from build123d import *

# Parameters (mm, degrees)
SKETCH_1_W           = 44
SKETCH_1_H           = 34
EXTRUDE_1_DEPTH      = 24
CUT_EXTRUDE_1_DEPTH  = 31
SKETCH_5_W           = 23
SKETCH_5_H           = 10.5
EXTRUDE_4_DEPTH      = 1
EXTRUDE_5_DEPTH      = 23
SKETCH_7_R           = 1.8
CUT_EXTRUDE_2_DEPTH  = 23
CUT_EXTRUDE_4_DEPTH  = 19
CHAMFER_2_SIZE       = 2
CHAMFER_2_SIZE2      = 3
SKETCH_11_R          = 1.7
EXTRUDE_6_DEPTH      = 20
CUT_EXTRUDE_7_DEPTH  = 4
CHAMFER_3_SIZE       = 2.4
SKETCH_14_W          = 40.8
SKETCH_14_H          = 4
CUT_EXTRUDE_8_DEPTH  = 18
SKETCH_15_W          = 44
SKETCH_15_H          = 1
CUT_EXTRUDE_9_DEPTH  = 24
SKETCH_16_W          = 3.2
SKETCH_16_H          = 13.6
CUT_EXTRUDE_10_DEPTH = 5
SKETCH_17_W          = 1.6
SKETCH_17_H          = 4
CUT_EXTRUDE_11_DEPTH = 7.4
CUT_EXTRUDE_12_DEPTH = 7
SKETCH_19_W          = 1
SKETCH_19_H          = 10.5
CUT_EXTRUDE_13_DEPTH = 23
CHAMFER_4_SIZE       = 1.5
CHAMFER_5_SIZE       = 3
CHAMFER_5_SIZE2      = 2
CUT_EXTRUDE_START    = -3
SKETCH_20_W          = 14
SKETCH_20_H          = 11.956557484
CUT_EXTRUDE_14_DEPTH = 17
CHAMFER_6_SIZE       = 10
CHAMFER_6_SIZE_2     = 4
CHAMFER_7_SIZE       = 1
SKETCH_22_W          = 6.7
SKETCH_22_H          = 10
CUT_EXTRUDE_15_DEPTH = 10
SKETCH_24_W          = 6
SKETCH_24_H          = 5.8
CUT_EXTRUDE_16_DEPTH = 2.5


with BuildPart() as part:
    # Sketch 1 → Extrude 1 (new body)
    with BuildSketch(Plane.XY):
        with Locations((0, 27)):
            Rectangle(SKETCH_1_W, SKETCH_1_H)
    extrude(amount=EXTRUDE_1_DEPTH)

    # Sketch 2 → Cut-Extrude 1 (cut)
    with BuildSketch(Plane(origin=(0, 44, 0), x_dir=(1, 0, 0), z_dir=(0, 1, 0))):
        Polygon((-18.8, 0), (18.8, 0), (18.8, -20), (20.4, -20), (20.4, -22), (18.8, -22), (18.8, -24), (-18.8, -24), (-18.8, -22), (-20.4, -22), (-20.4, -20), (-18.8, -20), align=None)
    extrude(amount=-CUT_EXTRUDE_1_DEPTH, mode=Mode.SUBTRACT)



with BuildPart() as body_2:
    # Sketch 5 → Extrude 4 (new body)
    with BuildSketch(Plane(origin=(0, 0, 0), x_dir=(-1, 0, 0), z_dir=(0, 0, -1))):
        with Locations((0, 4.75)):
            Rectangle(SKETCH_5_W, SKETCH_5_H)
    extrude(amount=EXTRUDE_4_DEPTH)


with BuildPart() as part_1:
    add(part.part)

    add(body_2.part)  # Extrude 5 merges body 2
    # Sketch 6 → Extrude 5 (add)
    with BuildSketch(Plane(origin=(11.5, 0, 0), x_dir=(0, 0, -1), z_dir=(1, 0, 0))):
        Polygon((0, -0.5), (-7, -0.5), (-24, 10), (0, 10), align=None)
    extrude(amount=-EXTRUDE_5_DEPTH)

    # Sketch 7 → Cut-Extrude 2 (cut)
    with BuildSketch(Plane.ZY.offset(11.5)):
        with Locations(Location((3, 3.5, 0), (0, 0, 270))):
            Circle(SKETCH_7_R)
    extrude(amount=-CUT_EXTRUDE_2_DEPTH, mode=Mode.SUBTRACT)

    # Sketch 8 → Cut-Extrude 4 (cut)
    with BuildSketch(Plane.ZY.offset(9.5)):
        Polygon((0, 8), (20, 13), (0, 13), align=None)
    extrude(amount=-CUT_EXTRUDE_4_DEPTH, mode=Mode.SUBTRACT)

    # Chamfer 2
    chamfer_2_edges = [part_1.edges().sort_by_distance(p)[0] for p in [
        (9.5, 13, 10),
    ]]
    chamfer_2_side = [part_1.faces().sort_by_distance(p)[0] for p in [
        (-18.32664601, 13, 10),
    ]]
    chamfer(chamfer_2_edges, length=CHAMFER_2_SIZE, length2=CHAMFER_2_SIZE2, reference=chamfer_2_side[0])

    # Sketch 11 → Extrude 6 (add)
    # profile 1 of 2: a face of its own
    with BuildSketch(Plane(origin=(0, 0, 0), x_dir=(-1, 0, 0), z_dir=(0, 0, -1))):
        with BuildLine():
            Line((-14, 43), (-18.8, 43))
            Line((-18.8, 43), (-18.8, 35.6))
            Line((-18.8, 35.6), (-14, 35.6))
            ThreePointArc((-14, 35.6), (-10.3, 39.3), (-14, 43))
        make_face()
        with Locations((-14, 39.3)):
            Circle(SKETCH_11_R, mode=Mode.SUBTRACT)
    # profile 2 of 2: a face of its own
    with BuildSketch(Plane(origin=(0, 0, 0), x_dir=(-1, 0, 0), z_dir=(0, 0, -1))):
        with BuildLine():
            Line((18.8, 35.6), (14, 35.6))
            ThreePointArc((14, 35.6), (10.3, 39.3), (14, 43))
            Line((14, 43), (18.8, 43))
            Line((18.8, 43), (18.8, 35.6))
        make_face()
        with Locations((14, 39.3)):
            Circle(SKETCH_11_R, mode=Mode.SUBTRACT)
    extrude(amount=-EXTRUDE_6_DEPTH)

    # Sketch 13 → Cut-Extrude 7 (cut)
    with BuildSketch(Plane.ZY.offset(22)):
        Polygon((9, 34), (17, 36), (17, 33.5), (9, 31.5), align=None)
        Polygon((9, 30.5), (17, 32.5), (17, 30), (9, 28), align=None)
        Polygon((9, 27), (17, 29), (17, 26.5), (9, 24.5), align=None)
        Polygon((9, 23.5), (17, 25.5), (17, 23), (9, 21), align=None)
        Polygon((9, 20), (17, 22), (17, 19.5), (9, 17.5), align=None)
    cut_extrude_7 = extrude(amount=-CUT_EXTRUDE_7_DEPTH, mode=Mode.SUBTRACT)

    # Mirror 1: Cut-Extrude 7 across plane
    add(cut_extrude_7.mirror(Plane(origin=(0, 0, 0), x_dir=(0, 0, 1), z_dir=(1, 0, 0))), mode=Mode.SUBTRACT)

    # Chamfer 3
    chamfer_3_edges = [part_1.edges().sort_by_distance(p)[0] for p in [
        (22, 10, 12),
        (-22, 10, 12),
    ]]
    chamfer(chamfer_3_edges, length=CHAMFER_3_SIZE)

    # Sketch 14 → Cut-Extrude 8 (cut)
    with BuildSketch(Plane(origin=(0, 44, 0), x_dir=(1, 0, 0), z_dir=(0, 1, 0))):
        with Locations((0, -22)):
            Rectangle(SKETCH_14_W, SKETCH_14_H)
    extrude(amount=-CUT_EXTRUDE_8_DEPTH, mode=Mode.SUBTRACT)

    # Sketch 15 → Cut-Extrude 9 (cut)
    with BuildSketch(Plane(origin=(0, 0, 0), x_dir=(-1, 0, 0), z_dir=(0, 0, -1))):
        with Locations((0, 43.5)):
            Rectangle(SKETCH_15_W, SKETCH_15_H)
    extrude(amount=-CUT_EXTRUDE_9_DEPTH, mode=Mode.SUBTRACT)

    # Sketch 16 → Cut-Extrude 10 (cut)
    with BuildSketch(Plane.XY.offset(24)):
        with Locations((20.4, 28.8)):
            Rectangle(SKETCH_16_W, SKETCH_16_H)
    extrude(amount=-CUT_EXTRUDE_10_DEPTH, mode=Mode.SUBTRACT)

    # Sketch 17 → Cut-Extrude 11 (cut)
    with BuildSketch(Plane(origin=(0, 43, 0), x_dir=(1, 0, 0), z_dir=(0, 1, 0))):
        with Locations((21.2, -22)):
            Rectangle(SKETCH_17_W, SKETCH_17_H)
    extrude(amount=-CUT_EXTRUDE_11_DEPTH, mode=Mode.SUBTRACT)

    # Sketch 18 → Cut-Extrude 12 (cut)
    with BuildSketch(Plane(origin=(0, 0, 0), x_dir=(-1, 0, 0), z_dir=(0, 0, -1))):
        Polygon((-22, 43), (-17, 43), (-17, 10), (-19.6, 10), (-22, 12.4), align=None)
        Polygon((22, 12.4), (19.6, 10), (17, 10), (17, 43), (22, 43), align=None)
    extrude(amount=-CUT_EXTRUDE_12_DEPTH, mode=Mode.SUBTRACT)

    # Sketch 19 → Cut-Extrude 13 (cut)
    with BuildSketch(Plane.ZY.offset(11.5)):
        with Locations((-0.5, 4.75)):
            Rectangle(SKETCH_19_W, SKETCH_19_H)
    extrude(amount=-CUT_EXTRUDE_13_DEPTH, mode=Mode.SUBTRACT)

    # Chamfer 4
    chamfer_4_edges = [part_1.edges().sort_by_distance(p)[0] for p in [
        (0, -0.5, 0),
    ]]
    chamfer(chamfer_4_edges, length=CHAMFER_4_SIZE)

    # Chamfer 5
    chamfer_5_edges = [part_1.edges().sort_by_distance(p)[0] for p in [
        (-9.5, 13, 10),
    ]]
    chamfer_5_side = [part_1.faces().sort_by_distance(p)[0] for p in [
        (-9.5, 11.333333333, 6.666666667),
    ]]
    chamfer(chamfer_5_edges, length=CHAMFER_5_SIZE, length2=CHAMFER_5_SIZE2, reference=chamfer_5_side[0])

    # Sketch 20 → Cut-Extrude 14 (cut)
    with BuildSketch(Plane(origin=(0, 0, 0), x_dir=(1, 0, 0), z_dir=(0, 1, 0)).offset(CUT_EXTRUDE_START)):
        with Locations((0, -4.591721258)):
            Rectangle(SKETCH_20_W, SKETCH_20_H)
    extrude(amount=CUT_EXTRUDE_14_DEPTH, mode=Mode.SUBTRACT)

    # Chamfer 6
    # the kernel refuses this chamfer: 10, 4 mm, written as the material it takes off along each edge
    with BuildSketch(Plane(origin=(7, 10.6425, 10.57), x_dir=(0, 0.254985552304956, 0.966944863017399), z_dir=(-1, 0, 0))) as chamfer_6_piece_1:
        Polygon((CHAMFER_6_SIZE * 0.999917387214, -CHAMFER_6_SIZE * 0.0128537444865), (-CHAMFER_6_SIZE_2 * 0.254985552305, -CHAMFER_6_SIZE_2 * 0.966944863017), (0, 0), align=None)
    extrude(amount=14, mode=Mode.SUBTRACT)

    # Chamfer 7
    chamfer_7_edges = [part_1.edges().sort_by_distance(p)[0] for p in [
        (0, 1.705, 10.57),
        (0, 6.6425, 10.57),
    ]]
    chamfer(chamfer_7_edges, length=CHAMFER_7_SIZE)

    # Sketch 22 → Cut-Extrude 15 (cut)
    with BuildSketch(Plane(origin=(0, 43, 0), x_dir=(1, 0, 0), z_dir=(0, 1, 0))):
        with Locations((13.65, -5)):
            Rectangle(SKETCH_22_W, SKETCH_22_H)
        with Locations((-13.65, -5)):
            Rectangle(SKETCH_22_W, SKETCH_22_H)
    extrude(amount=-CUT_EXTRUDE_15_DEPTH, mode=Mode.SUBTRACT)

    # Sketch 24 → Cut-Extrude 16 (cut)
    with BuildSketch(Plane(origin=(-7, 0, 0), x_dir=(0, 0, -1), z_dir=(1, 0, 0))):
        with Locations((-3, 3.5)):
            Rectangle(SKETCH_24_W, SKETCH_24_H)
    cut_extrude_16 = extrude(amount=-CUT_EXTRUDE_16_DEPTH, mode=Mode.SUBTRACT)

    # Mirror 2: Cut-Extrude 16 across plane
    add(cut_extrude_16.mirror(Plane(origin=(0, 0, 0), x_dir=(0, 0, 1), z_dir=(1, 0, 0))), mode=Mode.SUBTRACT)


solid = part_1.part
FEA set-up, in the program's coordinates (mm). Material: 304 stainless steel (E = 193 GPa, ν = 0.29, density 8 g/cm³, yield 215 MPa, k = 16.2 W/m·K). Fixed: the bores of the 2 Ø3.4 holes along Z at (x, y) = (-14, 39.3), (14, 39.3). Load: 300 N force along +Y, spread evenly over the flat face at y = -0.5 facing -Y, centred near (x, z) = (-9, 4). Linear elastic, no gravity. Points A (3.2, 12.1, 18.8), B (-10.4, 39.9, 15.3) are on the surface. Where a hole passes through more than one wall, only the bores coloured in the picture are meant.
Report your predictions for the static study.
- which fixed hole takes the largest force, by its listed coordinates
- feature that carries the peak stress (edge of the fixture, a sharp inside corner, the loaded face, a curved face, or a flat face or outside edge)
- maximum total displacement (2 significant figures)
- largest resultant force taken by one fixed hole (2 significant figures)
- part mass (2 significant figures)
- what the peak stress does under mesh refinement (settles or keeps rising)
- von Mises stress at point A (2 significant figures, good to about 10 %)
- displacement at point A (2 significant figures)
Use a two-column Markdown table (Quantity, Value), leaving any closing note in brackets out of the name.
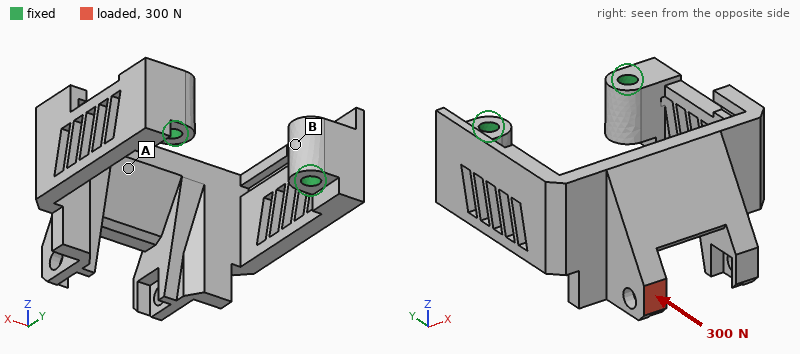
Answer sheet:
| Quantity | Value |
|---|---|
| which fixed hole takes the largest force, by its listed coordinates | (-14, 39.3) |
| feature that carries the peak stress | a sharp inside corner |
| maximum total displacement | 61 µm |
| largest resultant force taken by one fixed hole | 220 N |
| part mass | 55 g |
| what the peak stress does under mesh refinement | keeps rising |
| von Mises stress at point A | 25 MPa |
| displacement at point A | 15 µm |
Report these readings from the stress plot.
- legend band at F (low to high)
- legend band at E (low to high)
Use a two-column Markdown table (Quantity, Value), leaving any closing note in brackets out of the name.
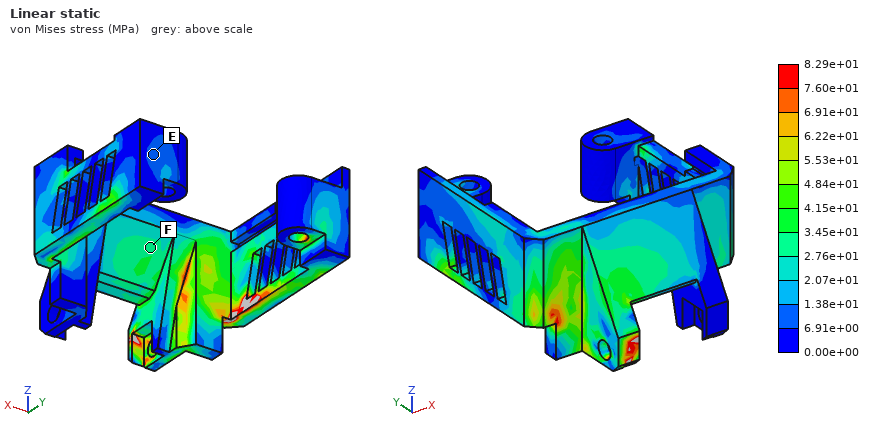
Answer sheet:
| Quantity | Value |
|---|---|
| legend band at F | 2.76e+01 to 3.45e+01 MPa |
| legend band at E | 6.91e+00 to 1.38e+01 MPa |
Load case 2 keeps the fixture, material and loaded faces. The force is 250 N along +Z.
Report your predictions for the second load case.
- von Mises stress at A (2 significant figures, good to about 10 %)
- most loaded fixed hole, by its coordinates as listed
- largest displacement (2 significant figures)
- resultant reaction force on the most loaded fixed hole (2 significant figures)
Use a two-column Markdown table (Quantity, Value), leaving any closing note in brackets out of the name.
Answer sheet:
| Quantity | Value |
|---|---|
| von Mises stress at A | 19 MPa |
| most loaded fixed hole, by its coordinates as listed | (-14, 39.3) |
| largest displacement | 91 µm |
| resultant reaction force on the most loaded fixed hole | 180 N |
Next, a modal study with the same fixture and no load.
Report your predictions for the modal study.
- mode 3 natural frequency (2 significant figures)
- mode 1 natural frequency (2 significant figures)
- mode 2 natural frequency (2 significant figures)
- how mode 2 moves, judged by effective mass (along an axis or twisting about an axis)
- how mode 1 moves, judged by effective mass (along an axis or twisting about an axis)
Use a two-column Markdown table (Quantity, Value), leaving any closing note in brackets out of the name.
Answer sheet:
| Quantity | Value |
|---|---|
| mode 3 natural frequency | 3600 Hz |
| mode 1 natural frequency | 1700 Hz |
| mode 2 natural frequency | 1900 Hz |
| how mode 2 moves, judged by effective mass | along Z |
| how mode 1 moves, judged by effective mass | along X |
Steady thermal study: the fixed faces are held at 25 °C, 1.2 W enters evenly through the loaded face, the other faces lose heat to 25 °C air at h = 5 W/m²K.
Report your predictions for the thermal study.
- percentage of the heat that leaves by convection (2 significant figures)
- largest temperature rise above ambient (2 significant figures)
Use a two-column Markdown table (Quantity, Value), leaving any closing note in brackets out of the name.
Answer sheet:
| Quantity | Value |
|---|---|
| percentage of the heat that leaves by convection | 48 % |
| largest temperature rise above ambient | 72 K |
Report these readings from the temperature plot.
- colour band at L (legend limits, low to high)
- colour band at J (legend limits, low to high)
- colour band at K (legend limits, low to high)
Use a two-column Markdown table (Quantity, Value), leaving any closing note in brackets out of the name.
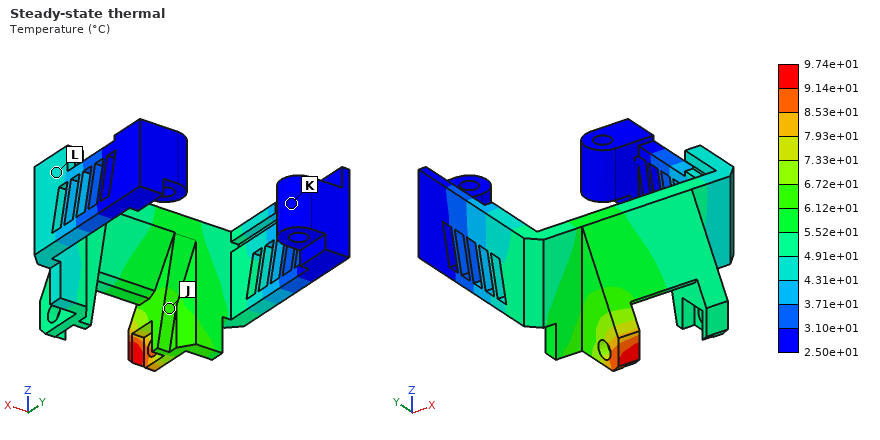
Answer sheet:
| Quantity | Value |
|---|---|
| colour band at L | 4.31e+01 to 4.91e+01 °C |
| colour band at J | 6.12e+01 to 6.72e+01 °C |
| colour band at K | 2.50e+01 to 3.10e+01 °C |
